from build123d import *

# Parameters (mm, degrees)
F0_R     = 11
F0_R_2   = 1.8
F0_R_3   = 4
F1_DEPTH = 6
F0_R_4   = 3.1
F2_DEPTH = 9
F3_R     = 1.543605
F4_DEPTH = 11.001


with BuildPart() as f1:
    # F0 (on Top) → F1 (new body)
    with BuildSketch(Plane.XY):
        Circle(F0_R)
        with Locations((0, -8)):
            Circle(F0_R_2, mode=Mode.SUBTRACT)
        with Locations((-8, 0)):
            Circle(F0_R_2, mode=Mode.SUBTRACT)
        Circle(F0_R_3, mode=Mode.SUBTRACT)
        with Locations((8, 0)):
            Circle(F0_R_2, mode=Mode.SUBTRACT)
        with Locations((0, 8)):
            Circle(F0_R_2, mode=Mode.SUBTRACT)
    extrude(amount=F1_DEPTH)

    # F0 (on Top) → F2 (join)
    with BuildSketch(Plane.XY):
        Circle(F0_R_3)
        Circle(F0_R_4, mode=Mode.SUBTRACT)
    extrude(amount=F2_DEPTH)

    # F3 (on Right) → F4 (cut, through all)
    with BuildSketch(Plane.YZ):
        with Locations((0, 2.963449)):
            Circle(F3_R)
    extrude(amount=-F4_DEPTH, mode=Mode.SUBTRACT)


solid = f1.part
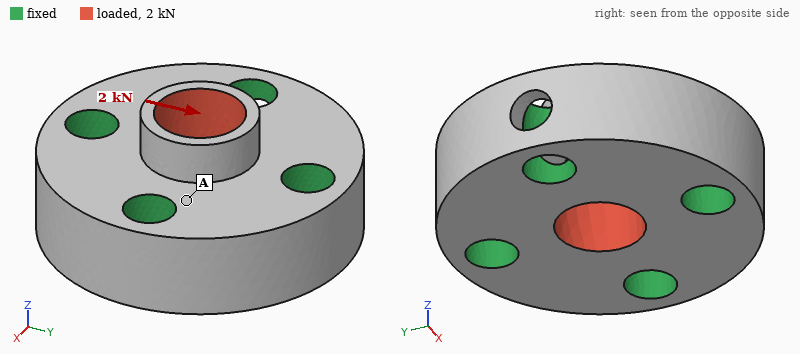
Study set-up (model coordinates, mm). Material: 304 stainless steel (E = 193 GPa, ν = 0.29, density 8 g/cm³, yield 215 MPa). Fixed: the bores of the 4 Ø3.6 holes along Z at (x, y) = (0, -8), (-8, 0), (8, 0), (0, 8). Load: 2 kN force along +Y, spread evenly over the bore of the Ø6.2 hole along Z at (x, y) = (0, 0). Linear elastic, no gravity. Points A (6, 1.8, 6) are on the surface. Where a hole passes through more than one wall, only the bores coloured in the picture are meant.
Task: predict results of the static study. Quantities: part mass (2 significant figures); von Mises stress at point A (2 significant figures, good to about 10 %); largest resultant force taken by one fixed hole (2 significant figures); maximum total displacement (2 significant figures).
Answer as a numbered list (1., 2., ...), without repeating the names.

1. 15 g
2. 14 MPa
3. 690 N
4. 3.4 µm
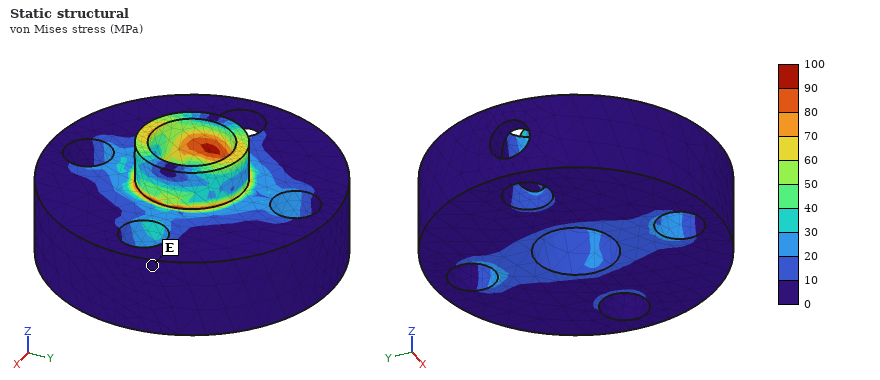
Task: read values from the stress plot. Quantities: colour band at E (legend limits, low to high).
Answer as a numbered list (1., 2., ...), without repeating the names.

1. 0 to 10 MPa
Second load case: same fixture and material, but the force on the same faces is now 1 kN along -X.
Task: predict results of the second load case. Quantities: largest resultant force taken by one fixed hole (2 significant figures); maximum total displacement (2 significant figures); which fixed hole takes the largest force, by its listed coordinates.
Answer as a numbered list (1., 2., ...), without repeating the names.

1. 350 N
2. 1.8 µm
3. (8, 0)
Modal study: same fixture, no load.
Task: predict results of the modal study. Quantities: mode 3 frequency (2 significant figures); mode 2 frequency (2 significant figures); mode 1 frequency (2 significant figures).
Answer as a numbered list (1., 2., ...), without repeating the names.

1. 110 kHz
2. 110 kHz
3. 110 kHz
